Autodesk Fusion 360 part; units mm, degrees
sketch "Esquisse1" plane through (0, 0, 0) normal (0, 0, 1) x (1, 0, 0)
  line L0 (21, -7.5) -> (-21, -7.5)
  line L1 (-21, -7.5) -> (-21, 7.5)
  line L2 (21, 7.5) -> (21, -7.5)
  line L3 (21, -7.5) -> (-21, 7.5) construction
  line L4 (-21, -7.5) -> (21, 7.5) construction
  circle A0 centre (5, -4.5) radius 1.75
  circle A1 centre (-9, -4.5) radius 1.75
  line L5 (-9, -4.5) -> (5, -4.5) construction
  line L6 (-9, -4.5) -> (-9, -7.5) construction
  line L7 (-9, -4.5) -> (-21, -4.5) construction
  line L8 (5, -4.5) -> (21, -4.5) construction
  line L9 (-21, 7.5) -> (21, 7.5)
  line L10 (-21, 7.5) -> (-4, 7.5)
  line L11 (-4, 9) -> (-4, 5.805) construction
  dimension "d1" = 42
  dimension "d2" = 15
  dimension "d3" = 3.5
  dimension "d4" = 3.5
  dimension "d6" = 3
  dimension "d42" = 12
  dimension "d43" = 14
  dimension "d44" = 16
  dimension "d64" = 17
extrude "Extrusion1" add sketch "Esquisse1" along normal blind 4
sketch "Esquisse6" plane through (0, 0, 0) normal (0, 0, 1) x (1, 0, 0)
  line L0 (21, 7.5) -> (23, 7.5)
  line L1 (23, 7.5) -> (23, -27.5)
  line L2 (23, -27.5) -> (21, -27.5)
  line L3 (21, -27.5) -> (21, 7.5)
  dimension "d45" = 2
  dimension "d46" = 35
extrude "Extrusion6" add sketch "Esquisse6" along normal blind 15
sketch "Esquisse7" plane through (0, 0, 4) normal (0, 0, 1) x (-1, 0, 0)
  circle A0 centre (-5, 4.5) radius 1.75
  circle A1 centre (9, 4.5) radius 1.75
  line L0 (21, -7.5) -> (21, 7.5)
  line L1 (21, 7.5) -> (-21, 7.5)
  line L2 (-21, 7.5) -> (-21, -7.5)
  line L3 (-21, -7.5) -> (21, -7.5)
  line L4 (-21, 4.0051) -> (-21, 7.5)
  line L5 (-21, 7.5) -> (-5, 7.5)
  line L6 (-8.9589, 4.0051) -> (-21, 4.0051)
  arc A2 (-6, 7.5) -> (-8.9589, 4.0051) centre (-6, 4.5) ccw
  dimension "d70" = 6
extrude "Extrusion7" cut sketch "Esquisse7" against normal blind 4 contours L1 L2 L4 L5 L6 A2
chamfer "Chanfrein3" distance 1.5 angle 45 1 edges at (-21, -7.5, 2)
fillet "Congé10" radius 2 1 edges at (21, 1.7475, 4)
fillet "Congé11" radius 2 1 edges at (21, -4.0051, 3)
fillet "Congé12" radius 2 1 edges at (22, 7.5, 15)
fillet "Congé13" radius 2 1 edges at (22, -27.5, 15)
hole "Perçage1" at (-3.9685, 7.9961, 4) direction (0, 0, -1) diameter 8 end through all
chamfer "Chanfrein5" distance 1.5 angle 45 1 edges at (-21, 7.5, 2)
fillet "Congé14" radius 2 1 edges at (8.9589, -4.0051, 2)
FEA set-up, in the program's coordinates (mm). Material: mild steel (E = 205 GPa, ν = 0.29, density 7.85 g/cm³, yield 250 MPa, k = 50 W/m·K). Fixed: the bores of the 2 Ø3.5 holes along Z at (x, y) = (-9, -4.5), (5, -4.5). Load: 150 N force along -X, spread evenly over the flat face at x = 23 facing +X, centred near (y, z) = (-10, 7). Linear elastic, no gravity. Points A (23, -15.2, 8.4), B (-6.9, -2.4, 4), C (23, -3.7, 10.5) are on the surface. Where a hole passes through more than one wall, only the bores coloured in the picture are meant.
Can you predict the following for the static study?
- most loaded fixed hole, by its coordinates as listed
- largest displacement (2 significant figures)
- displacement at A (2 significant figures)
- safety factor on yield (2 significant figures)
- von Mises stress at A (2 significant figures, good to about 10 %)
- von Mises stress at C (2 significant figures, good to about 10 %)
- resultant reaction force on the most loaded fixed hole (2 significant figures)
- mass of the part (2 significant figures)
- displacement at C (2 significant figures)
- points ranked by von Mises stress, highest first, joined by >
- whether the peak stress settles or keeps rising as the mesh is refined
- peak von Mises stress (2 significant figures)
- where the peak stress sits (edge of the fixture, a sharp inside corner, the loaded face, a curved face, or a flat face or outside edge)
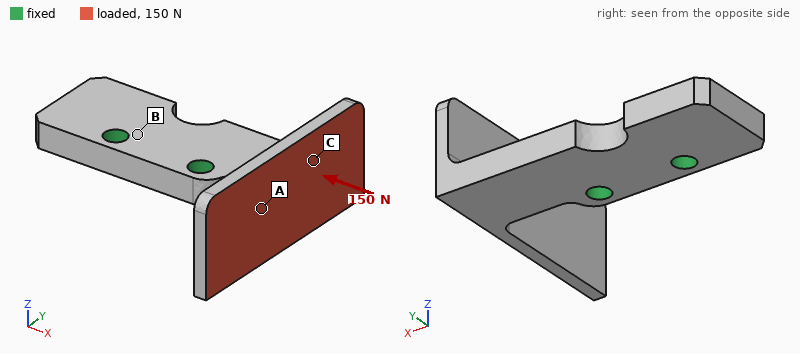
(5, -4.5)
0.14 mm
0.059 mm
0.89
30 MPa
70 MPa
200 N
25 g
0.022 mm
C > A > B
settles
280 MPa
a curved face
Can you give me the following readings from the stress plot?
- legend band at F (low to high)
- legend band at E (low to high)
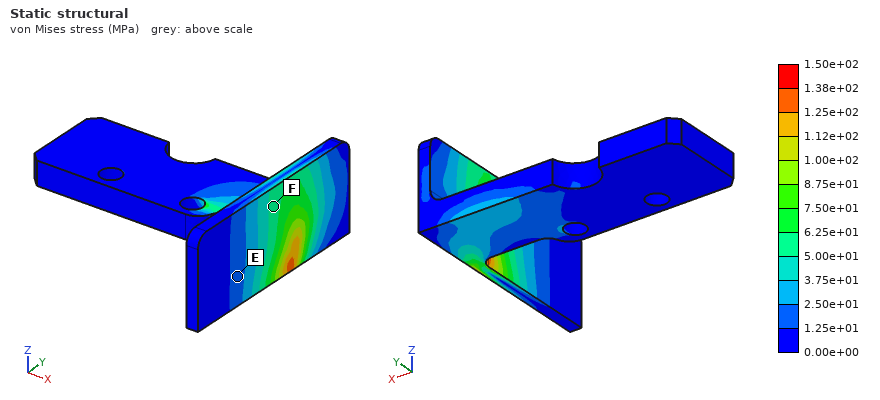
5.00e+01 to 6.25e+01 MPa
1.25e+01 to 2.50e+01 MPa
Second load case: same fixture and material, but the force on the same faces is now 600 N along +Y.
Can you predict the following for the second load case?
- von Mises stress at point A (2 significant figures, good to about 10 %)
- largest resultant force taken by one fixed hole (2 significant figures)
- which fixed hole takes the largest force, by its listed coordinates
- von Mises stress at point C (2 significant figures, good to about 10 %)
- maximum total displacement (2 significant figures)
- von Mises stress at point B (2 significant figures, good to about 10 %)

27 MPa
1.3 kN
(5, -4.5)
44 MPa
0.14 mm
20 MPa
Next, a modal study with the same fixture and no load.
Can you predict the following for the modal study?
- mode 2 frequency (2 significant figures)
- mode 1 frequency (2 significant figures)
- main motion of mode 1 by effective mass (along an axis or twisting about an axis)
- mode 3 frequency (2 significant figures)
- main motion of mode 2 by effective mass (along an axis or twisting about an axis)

2900 Hz
2300 Hz
along X
4800 Hz
along Z
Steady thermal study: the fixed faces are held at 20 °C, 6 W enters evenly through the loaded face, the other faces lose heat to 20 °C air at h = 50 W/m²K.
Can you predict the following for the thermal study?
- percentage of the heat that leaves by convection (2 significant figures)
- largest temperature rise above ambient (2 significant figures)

36 %
62 K
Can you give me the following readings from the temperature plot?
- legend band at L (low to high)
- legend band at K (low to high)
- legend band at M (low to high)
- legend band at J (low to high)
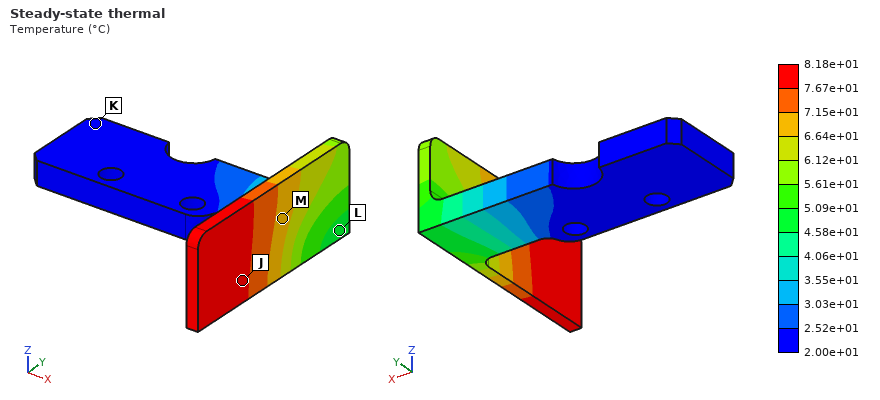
4.58e+01 to 5.09e+01 °C
2.00e+01 to 2.52e+01 °C
6.64e+01 to 7.15e+01 °C
7.67e+01 to 8.18e+01 °C
